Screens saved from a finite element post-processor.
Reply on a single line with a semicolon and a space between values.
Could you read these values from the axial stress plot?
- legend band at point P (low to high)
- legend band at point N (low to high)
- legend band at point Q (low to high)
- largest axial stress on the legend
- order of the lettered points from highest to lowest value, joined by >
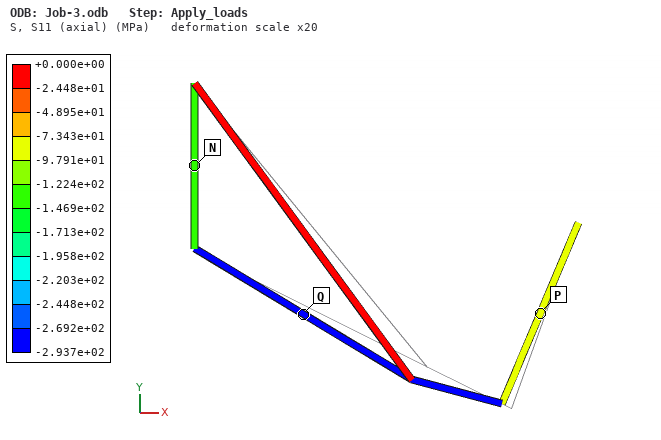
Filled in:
-9.791e+01 to -7.343e+01 MPa; -1.469e+02 to -1.224e+02 MPa; -2.937e+02 to -2.692e+02 MPa; +0.000e+00 MPa; P > N > Q
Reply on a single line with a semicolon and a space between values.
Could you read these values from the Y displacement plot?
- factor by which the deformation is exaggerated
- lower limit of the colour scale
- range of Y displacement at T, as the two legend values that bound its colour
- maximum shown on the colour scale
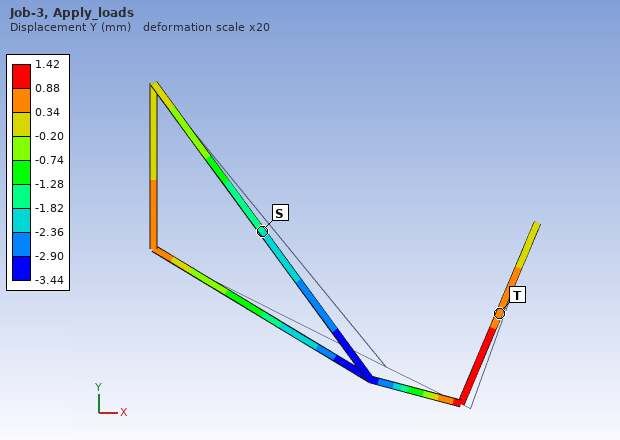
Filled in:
20; -3.44 mm; 0.34 to 0.88 mm; 1.42 mm
